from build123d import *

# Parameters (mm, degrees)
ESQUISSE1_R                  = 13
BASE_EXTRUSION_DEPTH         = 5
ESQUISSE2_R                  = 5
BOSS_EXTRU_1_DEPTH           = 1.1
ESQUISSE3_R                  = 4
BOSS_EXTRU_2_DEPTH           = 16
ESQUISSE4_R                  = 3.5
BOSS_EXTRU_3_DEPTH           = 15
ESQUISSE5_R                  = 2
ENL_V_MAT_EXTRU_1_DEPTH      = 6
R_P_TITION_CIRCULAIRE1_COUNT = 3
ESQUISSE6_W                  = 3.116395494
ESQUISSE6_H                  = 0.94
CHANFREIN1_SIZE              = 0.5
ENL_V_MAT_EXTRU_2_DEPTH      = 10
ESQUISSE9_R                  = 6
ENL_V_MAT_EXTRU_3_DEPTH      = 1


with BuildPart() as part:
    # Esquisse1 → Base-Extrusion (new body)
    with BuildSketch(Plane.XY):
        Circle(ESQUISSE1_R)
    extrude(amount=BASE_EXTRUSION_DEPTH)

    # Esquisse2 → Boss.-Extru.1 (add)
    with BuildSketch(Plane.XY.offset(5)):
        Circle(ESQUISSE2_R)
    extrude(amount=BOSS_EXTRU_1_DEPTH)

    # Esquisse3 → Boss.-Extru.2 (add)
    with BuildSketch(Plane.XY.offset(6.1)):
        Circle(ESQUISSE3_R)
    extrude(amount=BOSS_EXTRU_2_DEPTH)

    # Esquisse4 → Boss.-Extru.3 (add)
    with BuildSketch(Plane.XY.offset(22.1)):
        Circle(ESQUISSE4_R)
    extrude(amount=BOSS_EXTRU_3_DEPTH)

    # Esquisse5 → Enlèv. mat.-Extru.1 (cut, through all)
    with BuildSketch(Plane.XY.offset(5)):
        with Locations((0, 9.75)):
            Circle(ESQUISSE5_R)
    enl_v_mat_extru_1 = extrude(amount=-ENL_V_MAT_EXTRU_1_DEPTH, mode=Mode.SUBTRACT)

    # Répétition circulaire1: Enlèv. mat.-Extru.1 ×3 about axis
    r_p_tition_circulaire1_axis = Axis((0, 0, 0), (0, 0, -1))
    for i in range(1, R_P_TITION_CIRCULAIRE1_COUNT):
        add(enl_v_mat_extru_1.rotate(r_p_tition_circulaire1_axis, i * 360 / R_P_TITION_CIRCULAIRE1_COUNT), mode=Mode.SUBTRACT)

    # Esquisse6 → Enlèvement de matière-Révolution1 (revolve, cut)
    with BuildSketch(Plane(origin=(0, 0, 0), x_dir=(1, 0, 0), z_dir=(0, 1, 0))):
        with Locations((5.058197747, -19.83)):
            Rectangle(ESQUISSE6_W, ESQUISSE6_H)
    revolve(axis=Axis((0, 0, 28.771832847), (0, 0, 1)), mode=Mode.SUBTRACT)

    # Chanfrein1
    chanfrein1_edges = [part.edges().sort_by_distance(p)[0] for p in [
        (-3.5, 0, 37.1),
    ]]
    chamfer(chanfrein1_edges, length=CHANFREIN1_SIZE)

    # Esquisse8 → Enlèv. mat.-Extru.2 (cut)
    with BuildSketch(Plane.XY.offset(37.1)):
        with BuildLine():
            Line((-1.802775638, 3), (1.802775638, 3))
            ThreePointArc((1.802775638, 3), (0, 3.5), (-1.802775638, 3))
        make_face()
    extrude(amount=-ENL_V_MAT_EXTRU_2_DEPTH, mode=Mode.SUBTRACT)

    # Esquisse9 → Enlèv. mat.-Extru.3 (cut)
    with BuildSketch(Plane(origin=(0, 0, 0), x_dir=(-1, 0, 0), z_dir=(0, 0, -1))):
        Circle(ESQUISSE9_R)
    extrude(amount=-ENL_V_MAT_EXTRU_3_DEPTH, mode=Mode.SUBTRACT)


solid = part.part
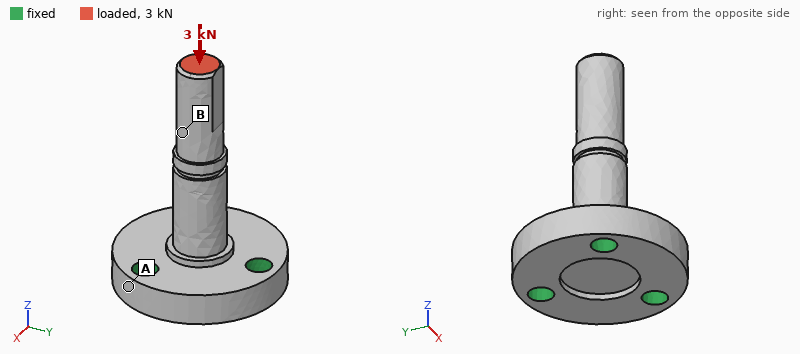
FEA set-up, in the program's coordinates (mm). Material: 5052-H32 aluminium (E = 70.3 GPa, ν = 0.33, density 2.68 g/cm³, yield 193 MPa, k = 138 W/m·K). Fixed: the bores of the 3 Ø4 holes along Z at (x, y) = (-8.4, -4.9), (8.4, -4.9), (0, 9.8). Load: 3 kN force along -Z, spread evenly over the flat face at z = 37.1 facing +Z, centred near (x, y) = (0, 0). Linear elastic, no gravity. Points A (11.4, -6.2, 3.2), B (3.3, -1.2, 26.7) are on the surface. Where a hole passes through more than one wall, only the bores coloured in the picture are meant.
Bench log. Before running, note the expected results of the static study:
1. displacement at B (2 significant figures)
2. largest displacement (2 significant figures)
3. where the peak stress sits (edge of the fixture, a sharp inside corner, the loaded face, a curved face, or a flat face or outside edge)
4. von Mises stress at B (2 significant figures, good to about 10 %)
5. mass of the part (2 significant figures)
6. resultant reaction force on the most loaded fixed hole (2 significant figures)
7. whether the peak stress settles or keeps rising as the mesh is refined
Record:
28 µm
41 µm
edge of the fixture
77 MPa
10 g
1.1 kN
keeps rising
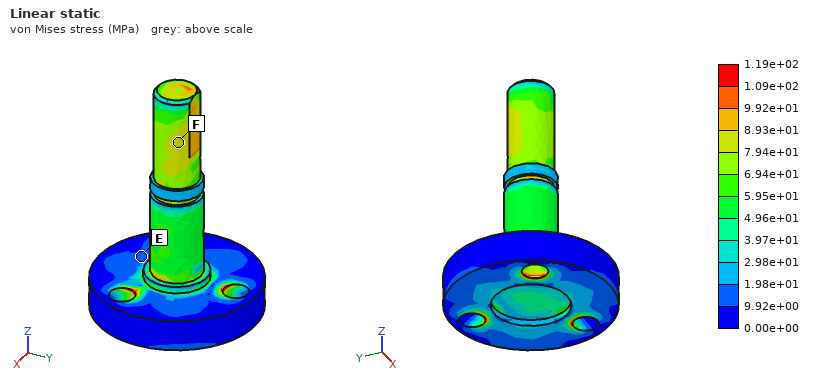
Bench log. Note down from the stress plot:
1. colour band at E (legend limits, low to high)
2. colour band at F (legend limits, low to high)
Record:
9.92e+00 to 1.98e+01 MPa
7.94e+01 to 8.93e+01 MPa
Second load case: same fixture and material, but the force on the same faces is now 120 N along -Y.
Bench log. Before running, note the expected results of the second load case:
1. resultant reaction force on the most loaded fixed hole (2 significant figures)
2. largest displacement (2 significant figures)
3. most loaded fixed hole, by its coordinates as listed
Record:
310 N
0.12 mm
(0, 9.8)
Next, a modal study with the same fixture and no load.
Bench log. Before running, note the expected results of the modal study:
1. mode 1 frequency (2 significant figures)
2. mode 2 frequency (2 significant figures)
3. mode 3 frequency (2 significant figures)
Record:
5600 Hz
5600 Hz
26 kHz
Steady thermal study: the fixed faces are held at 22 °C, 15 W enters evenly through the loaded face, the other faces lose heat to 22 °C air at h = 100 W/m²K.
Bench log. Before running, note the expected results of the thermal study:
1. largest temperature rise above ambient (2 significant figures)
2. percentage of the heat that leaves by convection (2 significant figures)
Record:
78 K
20 %
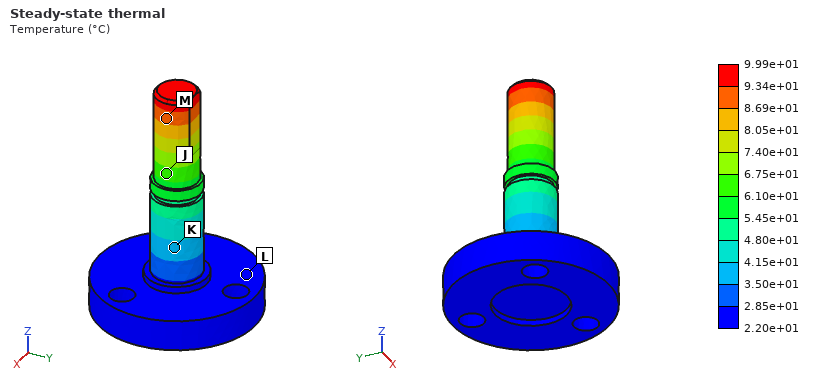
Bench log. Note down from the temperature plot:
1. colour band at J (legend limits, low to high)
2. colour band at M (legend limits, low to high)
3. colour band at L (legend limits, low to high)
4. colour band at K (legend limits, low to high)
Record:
6.10e+01 to 6.75e+01 °C
8.69e+01 to 9.34e+01 °C
2.20e+01 to 2.85e+01 °C
3.50e+01 to 4.15e+01 °C
